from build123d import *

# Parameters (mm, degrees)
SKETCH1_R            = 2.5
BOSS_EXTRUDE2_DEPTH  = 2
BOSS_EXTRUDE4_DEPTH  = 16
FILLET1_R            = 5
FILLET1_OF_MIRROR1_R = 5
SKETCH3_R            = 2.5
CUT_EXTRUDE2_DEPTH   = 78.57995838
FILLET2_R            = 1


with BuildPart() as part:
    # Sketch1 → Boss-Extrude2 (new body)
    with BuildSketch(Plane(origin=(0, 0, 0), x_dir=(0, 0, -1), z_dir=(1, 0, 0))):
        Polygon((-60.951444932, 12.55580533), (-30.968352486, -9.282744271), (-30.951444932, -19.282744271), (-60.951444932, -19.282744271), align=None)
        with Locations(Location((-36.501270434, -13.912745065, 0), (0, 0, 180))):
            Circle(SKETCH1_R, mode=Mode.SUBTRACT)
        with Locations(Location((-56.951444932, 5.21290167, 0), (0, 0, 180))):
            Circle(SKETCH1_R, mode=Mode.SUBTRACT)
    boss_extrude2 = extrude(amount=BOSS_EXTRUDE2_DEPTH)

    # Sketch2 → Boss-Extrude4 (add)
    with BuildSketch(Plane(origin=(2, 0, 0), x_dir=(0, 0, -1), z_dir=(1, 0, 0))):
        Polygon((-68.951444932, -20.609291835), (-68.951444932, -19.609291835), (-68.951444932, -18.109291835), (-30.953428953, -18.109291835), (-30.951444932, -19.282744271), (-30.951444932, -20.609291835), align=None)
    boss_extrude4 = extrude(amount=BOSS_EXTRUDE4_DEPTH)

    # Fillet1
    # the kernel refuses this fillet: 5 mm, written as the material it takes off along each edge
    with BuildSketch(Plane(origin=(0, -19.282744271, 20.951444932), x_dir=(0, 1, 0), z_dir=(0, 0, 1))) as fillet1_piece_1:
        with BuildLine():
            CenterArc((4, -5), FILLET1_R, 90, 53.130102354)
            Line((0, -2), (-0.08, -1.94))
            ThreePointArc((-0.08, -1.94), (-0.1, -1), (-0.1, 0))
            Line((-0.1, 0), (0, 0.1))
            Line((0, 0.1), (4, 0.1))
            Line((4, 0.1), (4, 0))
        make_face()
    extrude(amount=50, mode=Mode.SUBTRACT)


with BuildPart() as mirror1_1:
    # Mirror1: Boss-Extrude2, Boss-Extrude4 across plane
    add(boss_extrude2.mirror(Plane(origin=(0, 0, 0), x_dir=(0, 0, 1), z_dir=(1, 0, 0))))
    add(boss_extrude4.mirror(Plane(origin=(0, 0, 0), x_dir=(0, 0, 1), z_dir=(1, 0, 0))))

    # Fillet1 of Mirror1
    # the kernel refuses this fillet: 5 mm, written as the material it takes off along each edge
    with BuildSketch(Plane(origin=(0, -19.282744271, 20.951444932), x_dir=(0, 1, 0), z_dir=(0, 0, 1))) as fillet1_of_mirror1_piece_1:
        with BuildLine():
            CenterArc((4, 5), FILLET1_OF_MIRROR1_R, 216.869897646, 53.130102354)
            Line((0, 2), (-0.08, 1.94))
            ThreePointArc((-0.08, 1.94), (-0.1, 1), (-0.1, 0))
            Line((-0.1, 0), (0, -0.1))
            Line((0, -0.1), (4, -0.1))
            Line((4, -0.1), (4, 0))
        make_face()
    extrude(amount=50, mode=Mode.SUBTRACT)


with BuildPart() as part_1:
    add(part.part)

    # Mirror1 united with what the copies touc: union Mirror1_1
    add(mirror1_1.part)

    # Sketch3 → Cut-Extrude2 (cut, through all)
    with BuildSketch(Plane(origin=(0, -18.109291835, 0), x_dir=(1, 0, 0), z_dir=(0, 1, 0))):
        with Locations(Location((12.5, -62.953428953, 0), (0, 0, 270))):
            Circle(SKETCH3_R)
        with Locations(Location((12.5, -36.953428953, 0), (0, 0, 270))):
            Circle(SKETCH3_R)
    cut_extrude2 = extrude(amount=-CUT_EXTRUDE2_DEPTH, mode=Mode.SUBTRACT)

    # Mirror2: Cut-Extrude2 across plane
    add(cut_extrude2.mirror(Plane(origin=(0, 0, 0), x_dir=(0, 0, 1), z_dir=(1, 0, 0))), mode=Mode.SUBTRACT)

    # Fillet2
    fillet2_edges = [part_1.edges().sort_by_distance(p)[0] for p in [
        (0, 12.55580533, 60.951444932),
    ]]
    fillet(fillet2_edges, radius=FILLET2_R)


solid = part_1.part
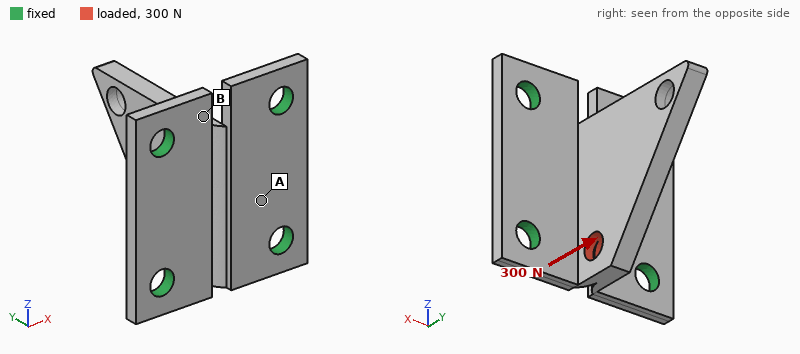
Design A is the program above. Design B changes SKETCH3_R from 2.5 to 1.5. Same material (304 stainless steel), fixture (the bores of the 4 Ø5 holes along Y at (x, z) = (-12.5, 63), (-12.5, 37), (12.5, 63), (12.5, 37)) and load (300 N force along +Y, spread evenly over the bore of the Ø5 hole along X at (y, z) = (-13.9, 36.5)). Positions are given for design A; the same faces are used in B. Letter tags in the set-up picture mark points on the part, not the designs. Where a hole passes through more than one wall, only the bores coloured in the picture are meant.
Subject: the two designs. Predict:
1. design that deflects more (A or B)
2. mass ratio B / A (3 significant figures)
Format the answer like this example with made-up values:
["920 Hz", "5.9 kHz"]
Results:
["B", "1.02"]
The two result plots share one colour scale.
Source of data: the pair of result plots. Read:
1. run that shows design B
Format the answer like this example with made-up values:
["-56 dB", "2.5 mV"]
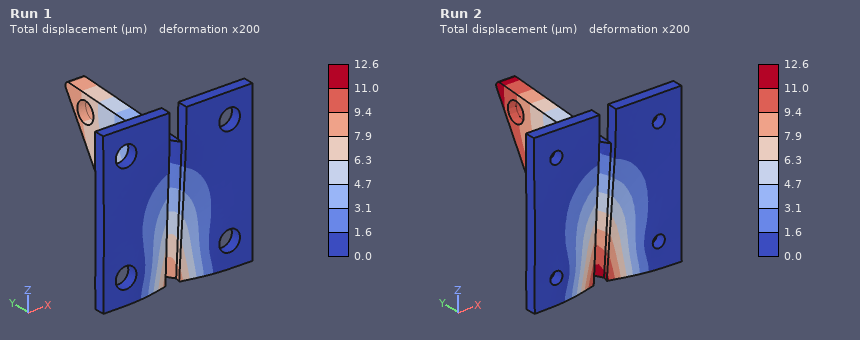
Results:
["Run 2"]
